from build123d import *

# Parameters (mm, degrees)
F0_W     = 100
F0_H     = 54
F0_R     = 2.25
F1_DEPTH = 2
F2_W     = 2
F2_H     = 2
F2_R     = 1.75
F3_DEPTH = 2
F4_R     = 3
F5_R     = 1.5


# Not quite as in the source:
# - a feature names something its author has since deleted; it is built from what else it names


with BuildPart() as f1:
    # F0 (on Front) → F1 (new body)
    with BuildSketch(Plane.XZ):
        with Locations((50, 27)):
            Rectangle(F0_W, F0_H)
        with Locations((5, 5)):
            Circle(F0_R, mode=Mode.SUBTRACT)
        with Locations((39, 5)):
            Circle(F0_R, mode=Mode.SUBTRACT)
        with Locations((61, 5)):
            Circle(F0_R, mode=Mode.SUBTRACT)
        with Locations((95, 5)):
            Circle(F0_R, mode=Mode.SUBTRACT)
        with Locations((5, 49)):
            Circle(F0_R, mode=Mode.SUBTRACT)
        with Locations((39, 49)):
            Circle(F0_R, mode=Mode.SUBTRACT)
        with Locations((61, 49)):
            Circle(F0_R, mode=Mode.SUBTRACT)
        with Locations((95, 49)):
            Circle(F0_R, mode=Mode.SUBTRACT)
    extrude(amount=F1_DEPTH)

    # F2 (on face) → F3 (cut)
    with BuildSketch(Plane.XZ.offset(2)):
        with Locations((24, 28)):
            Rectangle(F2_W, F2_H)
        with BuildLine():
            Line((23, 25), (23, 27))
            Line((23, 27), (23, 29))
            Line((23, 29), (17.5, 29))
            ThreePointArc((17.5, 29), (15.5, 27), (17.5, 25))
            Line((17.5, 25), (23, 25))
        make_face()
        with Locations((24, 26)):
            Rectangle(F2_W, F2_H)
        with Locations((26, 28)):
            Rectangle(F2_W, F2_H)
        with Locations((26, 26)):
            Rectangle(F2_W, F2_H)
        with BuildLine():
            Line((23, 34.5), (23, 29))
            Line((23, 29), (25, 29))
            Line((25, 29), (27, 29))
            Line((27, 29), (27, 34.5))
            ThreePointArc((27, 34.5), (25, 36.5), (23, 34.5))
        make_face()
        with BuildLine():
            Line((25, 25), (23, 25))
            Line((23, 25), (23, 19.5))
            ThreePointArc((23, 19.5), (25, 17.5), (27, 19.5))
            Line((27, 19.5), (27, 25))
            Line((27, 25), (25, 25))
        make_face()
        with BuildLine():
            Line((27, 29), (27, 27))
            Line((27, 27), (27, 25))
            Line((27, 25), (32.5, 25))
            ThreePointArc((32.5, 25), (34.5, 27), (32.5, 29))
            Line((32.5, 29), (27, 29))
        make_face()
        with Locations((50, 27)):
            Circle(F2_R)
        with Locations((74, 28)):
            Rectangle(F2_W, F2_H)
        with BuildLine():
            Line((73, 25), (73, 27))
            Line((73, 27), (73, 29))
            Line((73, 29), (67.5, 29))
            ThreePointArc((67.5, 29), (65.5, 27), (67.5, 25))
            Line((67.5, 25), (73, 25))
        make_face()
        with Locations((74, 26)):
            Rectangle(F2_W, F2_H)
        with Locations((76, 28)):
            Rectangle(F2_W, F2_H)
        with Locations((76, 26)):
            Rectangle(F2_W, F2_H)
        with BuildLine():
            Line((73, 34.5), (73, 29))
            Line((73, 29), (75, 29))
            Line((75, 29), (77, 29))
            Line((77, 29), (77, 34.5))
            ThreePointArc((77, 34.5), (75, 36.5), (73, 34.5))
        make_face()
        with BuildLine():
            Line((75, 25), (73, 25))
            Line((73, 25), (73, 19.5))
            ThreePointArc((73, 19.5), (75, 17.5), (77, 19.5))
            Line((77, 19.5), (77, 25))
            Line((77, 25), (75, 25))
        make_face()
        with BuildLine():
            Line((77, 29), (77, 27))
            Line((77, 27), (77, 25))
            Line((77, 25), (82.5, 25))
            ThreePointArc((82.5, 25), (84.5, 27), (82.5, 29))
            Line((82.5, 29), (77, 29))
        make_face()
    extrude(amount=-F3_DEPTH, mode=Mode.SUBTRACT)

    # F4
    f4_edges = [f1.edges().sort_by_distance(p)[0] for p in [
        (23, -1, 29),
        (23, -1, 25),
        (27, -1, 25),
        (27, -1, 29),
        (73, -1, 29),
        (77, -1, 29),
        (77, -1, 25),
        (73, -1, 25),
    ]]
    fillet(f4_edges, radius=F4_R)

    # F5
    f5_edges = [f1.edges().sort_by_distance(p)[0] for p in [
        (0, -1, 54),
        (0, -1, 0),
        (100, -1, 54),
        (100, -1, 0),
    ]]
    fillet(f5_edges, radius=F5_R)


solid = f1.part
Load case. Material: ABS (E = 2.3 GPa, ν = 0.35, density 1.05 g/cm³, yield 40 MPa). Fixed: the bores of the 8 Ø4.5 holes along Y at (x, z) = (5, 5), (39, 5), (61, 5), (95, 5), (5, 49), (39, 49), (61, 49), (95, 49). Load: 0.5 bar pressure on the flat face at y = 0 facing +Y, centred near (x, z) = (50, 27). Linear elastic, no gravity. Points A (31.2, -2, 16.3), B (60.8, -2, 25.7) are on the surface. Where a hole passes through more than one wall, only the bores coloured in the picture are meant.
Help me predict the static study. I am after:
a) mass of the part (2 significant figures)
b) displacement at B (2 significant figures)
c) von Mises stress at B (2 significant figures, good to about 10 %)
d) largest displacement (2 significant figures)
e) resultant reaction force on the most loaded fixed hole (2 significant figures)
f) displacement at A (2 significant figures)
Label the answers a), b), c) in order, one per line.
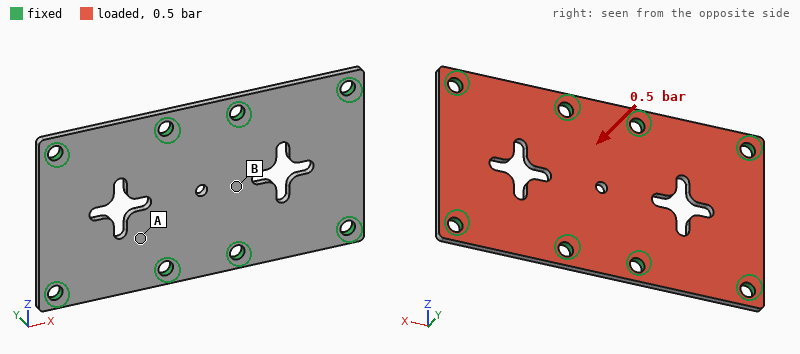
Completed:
a) 10 g
b) 0.34 mm
c) 7.2 MPa
d) 0.51 mm
e) 35 N
f) 0.26 mm
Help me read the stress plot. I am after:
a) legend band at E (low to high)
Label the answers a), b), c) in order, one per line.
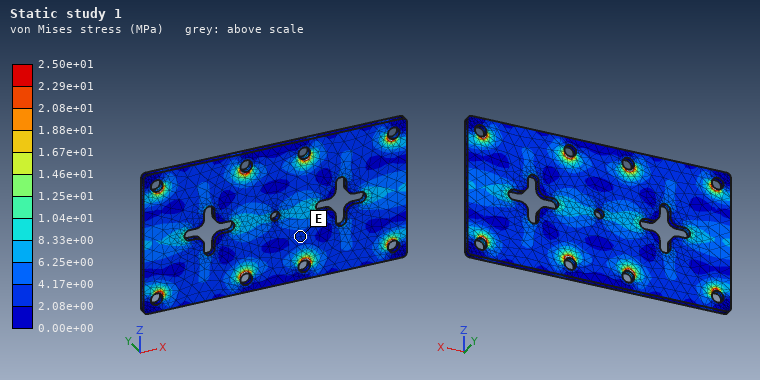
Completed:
a) 2.08e+00 to 4.17e+00 MPa
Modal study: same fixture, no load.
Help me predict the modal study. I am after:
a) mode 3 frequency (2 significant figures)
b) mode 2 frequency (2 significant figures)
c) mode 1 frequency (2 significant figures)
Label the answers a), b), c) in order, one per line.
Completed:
a) 1900 Hz
b) 1500 Hz
c) 1400 Hz
